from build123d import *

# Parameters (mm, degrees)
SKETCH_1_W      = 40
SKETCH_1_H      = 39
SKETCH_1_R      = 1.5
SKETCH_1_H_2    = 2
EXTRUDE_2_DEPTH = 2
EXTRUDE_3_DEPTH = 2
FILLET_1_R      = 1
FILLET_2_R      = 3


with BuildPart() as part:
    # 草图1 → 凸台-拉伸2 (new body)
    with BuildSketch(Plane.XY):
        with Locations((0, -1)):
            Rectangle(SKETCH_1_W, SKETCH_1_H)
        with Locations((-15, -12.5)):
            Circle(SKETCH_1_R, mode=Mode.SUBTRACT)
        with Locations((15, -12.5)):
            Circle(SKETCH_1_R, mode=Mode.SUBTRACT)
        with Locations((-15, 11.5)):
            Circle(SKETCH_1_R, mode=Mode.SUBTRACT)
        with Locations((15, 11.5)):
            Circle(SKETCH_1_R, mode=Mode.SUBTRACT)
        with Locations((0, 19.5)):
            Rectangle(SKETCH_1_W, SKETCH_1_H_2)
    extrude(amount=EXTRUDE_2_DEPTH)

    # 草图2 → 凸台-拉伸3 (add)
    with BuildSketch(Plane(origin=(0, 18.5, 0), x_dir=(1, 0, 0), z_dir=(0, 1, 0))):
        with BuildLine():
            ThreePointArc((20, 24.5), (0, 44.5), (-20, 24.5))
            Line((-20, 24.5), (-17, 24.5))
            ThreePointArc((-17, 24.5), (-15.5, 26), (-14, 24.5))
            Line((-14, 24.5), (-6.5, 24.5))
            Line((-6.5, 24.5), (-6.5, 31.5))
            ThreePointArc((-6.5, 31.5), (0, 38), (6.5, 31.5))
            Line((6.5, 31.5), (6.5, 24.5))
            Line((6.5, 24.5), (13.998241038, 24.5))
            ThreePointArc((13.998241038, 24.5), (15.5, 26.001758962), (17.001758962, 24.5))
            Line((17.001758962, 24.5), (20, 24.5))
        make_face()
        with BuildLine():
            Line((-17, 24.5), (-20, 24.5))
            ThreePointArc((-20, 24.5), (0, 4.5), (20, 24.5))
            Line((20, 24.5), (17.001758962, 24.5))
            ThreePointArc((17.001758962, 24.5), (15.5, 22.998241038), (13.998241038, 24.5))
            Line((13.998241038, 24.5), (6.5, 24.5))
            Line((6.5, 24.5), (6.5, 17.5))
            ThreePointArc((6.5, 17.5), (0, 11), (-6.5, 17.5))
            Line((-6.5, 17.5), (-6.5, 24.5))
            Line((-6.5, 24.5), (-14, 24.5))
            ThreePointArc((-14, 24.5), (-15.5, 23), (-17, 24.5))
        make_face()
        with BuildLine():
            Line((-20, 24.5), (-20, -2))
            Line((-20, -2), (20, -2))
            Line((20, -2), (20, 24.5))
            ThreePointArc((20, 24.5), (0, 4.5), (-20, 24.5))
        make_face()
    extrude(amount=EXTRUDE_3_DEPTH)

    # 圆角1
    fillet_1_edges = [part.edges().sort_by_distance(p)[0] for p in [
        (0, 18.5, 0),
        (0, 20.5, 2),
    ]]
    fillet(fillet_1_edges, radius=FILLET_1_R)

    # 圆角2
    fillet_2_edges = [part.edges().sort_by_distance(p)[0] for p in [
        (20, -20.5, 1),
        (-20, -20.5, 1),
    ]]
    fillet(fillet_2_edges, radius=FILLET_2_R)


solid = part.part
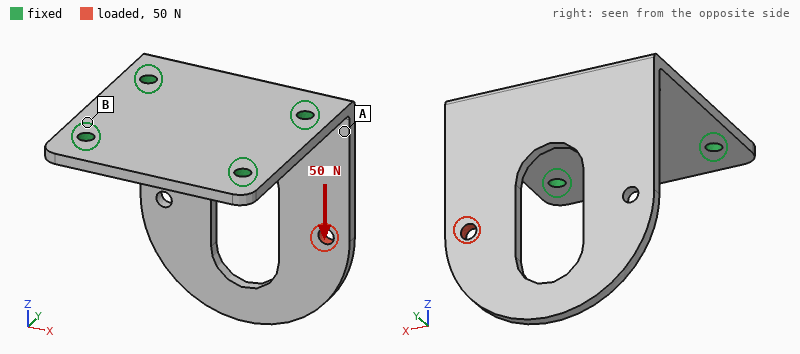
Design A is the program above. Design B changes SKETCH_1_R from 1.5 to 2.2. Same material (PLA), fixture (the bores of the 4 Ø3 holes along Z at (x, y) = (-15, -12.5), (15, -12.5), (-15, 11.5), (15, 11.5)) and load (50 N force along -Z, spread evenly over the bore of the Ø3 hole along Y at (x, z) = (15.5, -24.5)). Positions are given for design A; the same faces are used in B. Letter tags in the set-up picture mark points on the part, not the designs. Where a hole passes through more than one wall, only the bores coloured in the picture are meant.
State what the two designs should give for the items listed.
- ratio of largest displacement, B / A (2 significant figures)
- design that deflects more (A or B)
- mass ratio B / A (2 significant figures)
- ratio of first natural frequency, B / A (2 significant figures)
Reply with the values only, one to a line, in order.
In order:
0.79
A
0.99
1.0
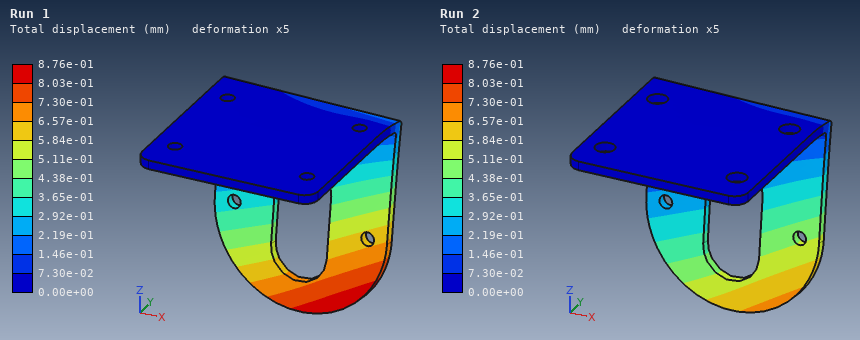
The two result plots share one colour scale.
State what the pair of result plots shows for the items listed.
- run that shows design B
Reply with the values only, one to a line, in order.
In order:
Run 2
